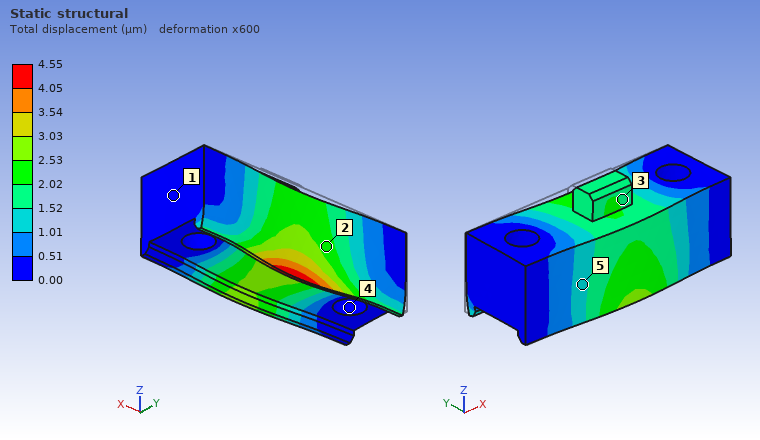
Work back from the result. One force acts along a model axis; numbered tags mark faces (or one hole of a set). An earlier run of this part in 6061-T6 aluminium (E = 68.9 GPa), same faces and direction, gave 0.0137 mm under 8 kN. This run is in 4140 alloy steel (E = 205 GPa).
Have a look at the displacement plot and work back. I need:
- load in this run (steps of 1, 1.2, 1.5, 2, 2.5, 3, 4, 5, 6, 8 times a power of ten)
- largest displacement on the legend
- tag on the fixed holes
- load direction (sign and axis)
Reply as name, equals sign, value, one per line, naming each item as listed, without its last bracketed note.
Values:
load in this run = 8 kN
largest displacement on the legend = 4.55 µm
tag on the fixed holes = 4
load direction = -Y
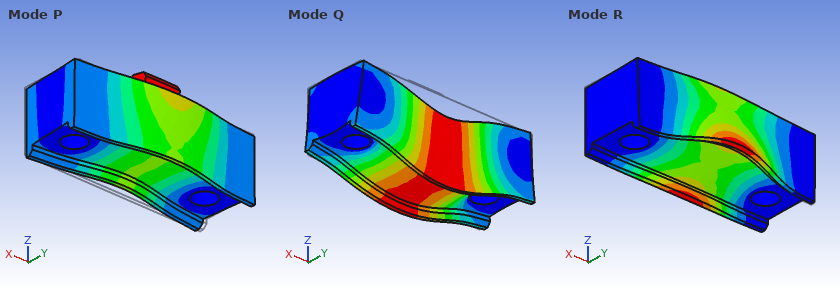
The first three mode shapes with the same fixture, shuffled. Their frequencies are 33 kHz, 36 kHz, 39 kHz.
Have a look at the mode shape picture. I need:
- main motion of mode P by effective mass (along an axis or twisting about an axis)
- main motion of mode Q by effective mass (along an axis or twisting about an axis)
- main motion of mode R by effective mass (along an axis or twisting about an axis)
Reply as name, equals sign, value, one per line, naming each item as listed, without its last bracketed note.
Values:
main motion of mode P by effective mass = along Y
main motion of mode Q by effective mass = along Z
main motion of mode R by effective mass = twisting about X
